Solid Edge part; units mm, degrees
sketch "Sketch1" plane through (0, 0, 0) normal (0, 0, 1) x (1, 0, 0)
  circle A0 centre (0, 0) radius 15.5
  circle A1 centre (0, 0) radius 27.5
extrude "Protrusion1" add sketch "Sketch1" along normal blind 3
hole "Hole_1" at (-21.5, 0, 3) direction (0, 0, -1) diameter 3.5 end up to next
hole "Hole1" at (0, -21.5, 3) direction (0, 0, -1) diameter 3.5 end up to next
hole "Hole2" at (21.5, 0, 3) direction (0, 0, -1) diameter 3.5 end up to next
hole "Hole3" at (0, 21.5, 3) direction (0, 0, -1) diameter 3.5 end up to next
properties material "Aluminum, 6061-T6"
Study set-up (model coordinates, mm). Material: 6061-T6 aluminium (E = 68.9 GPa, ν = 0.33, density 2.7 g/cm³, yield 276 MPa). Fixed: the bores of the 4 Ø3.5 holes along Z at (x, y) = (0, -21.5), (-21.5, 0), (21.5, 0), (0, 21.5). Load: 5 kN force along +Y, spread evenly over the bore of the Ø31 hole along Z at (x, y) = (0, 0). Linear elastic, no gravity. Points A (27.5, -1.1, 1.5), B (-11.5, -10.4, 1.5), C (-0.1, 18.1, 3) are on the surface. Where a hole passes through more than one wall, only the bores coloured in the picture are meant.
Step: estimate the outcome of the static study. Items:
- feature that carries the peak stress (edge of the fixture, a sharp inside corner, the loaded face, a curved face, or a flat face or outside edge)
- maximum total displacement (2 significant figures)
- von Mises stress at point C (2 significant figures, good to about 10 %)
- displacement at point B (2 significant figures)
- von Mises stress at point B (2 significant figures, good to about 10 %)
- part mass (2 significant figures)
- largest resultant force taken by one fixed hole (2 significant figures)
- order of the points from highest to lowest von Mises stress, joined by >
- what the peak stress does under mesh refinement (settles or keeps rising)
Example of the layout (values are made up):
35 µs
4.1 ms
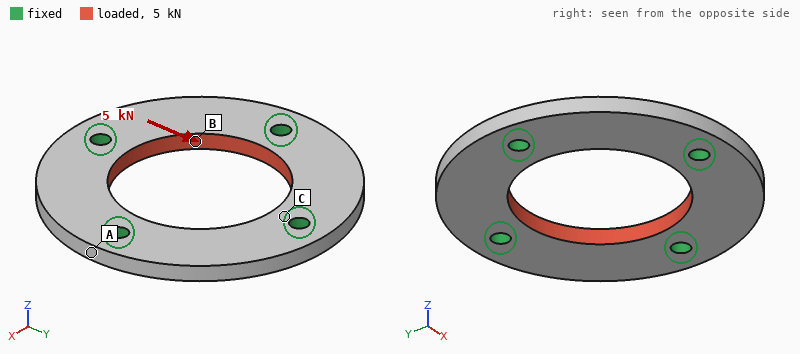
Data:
edge of the fixture
8.2 µm
39 MPa
8.2 µm
26 MPa
13 g
1.4 kN
C > B > A
keeps rising
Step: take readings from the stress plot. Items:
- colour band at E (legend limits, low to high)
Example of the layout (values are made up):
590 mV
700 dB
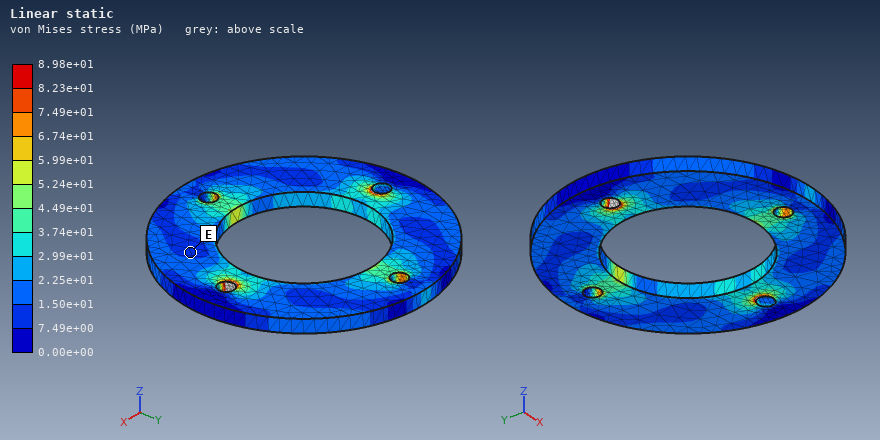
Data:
7.49e+00 to 1.50e+01 MPa
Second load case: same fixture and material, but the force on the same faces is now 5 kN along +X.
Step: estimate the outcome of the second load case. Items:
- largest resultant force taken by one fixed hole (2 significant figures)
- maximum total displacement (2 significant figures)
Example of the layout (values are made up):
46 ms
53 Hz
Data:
1.4 kN
8.2 µm
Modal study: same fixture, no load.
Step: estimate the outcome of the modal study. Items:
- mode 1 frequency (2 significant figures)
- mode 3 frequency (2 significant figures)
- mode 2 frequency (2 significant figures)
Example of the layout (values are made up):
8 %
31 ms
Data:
12 kHz
12 kHz
12 kHz
